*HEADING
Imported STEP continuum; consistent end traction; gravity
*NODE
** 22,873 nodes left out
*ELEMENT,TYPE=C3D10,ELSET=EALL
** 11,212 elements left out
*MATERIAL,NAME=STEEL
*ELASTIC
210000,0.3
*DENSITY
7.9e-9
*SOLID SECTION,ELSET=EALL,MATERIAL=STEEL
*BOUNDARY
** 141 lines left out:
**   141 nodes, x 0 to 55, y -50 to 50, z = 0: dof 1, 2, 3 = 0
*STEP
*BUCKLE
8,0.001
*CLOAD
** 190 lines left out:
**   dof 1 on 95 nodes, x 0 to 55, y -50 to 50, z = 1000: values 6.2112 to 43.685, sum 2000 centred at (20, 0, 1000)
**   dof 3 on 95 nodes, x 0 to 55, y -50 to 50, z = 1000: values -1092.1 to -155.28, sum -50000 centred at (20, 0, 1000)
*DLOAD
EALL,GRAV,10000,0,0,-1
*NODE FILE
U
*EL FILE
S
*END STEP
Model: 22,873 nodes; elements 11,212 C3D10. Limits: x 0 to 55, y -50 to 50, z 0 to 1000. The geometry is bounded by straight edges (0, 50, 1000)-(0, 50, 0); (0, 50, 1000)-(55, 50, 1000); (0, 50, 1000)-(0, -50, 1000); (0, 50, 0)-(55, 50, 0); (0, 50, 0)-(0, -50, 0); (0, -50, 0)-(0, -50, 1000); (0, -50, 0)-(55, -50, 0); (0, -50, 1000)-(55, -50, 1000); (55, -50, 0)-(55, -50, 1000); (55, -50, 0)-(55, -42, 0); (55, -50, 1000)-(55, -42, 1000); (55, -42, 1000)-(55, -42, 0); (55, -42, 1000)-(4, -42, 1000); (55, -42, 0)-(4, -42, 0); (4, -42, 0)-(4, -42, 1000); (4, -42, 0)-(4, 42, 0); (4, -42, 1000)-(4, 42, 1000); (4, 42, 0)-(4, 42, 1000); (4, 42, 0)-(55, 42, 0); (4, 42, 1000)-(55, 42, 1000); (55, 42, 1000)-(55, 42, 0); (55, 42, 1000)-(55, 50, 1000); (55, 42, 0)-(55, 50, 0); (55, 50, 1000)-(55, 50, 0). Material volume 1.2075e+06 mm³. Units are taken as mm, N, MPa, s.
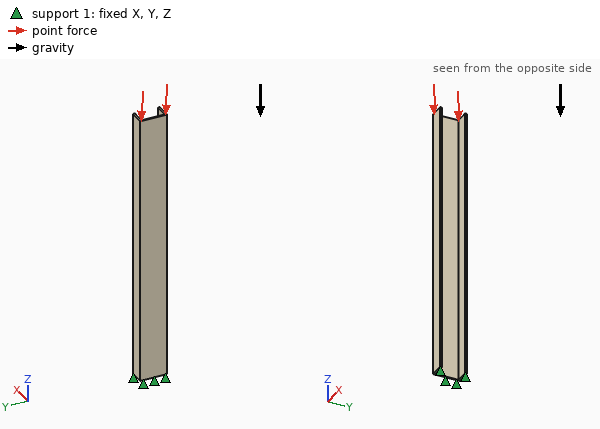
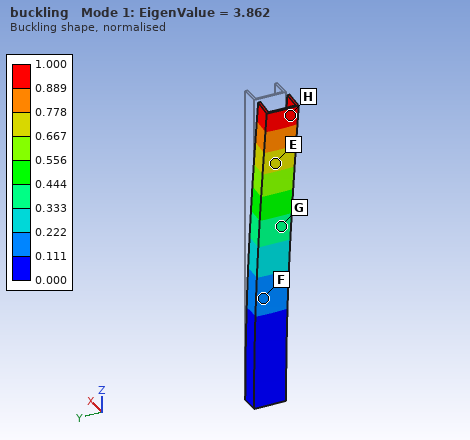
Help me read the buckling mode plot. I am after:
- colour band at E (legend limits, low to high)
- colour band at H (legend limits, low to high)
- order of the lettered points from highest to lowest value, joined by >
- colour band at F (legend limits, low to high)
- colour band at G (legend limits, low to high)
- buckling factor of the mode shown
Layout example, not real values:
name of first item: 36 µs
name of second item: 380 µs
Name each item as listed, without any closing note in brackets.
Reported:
colour band at E: 0.667 to 0.778
colour band at H: 0.889 to 1.000
order of the lettered points from highest to lowest value, joined by >: H > E > G > F
colour band at F: 0.111 to 0.222
colour band at G: 0.333 to 0.444
buckling factor of the mode shown: 3.862
